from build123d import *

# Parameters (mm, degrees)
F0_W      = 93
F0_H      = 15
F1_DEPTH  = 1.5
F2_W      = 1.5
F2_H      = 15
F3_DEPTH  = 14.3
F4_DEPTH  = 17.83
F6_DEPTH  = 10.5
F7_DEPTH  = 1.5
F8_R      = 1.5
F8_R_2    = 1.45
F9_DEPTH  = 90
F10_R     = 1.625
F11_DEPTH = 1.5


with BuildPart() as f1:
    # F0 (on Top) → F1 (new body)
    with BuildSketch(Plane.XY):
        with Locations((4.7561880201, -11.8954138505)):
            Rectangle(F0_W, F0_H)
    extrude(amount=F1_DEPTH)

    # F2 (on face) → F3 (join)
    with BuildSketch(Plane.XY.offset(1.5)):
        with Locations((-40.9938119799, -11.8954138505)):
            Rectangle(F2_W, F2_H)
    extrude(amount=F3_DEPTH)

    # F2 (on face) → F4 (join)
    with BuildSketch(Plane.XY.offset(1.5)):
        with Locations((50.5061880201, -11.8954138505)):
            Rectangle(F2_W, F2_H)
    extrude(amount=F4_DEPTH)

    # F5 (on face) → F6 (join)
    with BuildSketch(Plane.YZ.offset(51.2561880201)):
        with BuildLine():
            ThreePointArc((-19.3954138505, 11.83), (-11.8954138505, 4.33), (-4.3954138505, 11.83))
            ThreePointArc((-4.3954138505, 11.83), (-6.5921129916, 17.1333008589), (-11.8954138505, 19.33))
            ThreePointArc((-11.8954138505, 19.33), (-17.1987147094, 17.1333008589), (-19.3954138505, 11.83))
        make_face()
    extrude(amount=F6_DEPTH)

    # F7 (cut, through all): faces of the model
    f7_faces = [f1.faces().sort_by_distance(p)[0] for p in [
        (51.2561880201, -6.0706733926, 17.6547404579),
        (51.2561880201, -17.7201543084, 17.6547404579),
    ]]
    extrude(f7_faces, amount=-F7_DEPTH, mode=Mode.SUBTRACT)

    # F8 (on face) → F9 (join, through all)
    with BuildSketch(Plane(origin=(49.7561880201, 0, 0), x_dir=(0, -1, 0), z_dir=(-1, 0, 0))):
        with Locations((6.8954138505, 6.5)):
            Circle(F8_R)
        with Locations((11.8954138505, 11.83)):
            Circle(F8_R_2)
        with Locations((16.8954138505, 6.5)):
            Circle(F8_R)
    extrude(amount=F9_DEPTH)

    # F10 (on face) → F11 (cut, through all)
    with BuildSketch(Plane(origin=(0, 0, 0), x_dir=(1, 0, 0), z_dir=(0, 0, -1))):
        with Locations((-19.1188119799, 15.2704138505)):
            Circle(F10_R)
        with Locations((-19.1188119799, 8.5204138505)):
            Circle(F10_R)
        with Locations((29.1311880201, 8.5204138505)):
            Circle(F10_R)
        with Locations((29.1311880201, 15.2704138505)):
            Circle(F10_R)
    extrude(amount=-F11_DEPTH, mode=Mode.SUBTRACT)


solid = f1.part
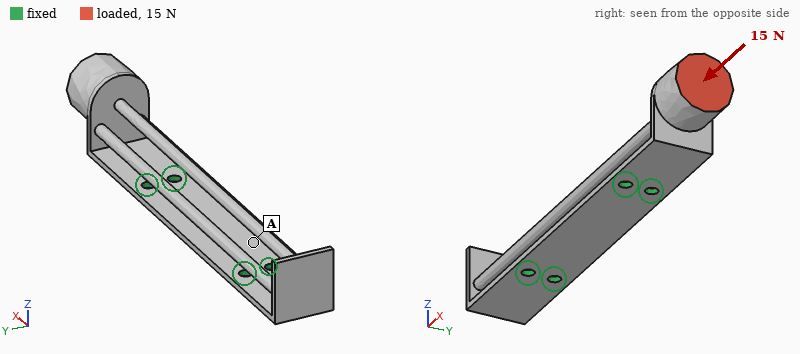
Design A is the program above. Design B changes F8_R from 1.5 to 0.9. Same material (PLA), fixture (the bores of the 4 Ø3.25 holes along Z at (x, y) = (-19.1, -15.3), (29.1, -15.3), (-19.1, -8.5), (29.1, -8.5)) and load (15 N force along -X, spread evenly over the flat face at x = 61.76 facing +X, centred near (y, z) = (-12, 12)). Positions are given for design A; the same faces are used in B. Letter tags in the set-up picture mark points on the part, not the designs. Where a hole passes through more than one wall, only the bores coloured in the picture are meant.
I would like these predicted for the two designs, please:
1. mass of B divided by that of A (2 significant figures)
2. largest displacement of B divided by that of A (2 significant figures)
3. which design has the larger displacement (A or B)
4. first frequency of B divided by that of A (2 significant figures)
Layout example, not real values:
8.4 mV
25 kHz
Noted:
0.87
1.6
B
0.89
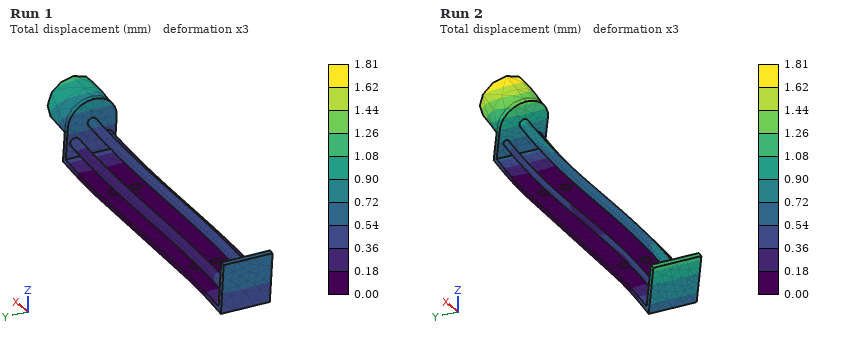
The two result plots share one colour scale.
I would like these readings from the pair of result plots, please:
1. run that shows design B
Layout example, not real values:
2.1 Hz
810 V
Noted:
Run 2
